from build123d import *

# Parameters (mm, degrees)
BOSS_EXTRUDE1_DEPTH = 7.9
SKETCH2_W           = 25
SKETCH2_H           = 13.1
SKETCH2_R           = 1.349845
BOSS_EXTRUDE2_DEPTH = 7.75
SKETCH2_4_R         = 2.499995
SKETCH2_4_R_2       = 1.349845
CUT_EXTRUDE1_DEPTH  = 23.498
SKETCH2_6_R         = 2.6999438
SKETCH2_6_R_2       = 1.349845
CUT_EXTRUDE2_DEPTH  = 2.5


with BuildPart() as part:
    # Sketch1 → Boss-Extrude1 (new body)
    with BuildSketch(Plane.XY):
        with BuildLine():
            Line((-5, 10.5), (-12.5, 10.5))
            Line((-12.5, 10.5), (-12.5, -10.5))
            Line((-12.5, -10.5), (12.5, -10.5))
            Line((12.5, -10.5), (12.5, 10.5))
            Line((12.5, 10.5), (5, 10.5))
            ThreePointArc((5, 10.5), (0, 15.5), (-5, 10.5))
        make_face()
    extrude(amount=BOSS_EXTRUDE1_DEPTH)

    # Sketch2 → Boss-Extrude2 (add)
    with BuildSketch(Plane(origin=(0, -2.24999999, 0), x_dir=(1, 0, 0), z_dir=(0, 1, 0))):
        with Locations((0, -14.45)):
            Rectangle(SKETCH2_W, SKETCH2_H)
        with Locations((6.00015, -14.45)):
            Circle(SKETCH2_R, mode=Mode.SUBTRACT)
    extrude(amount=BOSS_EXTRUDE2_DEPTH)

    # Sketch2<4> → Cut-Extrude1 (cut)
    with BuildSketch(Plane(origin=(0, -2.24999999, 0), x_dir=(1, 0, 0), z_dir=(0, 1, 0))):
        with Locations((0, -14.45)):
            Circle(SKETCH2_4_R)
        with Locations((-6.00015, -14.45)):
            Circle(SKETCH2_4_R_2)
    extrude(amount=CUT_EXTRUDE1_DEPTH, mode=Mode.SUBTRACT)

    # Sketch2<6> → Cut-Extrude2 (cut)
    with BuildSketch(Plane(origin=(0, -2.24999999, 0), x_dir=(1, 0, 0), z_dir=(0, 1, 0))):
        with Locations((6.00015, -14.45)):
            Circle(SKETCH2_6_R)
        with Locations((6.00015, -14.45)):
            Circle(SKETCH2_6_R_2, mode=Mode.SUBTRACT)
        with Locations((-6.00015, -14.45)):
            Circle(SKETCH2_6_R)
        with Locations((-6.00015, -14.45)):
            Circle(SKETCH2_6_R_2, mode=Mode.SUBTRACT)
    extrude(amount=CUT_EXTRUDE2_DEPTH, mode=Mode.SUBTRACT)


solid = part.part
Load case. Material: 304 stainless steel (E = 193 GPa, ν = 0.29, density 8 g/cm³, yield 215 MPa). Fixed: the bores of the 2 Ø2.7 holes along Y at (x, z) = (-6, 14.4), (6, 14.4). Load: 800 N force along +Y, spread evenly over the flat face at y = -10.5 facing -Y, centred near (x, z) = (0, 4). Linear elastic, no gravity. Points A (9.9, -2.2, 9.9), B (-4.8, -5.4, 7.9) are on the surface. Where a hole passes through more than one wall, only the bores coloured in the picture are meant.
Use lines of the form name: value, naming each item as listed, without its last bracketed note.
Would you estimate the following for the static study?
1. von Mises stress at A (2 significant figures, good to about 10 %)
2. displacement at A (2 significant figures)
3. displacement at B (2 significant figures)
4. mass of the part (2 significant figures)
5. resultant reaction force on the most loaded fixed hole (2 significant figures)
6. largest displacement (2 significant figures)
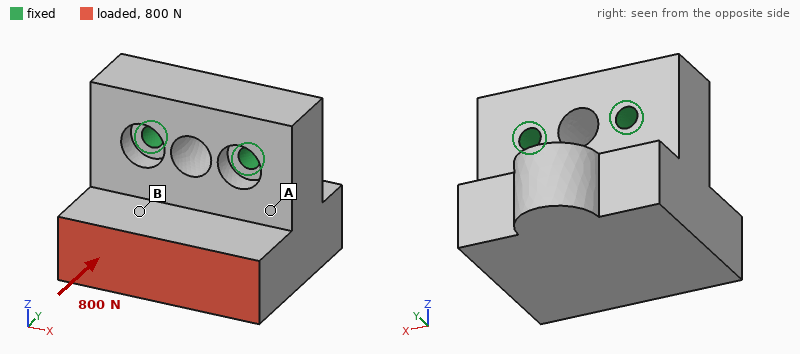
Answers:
von Mises stress at A: 21 MPa
displacement at A: 3.0 µm
displacement at B: 5.3 µm
mass of the part: 53 g
resultant reaction force on the most loaded fixed hole: 400 N
largest displacement: 11 µm
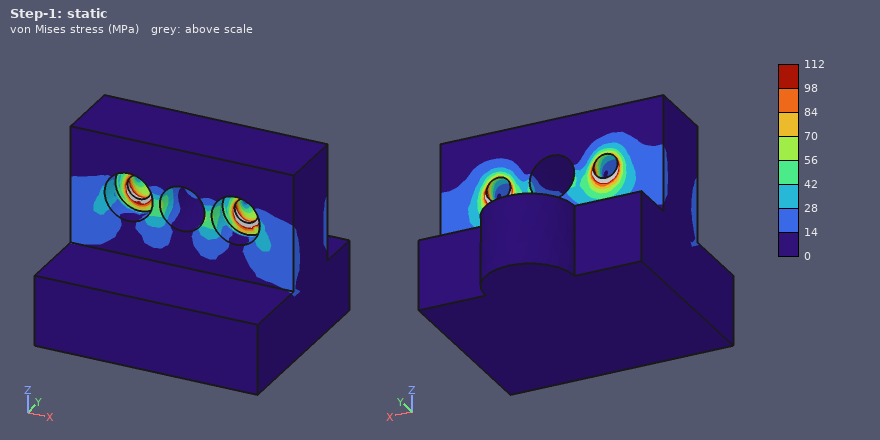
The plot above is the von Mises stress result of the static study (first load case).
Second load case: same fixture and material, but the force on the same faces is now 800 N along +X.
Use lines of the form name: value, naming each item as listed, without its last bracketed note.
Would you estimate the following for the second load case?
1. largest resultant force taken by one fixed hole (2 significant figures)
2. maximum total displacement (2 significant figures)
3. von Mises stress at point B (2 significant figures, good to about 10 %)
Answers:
largest resultant force taken by one fixed hole: 960 N
maximum total displacement: 6.5 µm
von Mises stress at point B: 17 MPa
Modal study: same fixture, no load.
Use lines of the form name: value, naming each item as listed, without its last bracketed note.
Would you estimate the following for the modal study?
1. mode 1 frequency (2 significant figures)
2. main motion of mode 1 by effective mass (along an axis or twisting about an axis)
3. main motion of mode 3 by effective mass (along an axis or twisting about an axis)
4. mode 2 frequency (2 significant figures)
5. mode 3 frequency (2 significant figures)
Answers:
mode 1 frequency: 8100 Hz
main motion of mode 1 by effective mass: along Y
main motion of mode 3 by effective mass: along X
mode 2 frequency: 16 kHz
mode 3 frequency: 19 kHz
